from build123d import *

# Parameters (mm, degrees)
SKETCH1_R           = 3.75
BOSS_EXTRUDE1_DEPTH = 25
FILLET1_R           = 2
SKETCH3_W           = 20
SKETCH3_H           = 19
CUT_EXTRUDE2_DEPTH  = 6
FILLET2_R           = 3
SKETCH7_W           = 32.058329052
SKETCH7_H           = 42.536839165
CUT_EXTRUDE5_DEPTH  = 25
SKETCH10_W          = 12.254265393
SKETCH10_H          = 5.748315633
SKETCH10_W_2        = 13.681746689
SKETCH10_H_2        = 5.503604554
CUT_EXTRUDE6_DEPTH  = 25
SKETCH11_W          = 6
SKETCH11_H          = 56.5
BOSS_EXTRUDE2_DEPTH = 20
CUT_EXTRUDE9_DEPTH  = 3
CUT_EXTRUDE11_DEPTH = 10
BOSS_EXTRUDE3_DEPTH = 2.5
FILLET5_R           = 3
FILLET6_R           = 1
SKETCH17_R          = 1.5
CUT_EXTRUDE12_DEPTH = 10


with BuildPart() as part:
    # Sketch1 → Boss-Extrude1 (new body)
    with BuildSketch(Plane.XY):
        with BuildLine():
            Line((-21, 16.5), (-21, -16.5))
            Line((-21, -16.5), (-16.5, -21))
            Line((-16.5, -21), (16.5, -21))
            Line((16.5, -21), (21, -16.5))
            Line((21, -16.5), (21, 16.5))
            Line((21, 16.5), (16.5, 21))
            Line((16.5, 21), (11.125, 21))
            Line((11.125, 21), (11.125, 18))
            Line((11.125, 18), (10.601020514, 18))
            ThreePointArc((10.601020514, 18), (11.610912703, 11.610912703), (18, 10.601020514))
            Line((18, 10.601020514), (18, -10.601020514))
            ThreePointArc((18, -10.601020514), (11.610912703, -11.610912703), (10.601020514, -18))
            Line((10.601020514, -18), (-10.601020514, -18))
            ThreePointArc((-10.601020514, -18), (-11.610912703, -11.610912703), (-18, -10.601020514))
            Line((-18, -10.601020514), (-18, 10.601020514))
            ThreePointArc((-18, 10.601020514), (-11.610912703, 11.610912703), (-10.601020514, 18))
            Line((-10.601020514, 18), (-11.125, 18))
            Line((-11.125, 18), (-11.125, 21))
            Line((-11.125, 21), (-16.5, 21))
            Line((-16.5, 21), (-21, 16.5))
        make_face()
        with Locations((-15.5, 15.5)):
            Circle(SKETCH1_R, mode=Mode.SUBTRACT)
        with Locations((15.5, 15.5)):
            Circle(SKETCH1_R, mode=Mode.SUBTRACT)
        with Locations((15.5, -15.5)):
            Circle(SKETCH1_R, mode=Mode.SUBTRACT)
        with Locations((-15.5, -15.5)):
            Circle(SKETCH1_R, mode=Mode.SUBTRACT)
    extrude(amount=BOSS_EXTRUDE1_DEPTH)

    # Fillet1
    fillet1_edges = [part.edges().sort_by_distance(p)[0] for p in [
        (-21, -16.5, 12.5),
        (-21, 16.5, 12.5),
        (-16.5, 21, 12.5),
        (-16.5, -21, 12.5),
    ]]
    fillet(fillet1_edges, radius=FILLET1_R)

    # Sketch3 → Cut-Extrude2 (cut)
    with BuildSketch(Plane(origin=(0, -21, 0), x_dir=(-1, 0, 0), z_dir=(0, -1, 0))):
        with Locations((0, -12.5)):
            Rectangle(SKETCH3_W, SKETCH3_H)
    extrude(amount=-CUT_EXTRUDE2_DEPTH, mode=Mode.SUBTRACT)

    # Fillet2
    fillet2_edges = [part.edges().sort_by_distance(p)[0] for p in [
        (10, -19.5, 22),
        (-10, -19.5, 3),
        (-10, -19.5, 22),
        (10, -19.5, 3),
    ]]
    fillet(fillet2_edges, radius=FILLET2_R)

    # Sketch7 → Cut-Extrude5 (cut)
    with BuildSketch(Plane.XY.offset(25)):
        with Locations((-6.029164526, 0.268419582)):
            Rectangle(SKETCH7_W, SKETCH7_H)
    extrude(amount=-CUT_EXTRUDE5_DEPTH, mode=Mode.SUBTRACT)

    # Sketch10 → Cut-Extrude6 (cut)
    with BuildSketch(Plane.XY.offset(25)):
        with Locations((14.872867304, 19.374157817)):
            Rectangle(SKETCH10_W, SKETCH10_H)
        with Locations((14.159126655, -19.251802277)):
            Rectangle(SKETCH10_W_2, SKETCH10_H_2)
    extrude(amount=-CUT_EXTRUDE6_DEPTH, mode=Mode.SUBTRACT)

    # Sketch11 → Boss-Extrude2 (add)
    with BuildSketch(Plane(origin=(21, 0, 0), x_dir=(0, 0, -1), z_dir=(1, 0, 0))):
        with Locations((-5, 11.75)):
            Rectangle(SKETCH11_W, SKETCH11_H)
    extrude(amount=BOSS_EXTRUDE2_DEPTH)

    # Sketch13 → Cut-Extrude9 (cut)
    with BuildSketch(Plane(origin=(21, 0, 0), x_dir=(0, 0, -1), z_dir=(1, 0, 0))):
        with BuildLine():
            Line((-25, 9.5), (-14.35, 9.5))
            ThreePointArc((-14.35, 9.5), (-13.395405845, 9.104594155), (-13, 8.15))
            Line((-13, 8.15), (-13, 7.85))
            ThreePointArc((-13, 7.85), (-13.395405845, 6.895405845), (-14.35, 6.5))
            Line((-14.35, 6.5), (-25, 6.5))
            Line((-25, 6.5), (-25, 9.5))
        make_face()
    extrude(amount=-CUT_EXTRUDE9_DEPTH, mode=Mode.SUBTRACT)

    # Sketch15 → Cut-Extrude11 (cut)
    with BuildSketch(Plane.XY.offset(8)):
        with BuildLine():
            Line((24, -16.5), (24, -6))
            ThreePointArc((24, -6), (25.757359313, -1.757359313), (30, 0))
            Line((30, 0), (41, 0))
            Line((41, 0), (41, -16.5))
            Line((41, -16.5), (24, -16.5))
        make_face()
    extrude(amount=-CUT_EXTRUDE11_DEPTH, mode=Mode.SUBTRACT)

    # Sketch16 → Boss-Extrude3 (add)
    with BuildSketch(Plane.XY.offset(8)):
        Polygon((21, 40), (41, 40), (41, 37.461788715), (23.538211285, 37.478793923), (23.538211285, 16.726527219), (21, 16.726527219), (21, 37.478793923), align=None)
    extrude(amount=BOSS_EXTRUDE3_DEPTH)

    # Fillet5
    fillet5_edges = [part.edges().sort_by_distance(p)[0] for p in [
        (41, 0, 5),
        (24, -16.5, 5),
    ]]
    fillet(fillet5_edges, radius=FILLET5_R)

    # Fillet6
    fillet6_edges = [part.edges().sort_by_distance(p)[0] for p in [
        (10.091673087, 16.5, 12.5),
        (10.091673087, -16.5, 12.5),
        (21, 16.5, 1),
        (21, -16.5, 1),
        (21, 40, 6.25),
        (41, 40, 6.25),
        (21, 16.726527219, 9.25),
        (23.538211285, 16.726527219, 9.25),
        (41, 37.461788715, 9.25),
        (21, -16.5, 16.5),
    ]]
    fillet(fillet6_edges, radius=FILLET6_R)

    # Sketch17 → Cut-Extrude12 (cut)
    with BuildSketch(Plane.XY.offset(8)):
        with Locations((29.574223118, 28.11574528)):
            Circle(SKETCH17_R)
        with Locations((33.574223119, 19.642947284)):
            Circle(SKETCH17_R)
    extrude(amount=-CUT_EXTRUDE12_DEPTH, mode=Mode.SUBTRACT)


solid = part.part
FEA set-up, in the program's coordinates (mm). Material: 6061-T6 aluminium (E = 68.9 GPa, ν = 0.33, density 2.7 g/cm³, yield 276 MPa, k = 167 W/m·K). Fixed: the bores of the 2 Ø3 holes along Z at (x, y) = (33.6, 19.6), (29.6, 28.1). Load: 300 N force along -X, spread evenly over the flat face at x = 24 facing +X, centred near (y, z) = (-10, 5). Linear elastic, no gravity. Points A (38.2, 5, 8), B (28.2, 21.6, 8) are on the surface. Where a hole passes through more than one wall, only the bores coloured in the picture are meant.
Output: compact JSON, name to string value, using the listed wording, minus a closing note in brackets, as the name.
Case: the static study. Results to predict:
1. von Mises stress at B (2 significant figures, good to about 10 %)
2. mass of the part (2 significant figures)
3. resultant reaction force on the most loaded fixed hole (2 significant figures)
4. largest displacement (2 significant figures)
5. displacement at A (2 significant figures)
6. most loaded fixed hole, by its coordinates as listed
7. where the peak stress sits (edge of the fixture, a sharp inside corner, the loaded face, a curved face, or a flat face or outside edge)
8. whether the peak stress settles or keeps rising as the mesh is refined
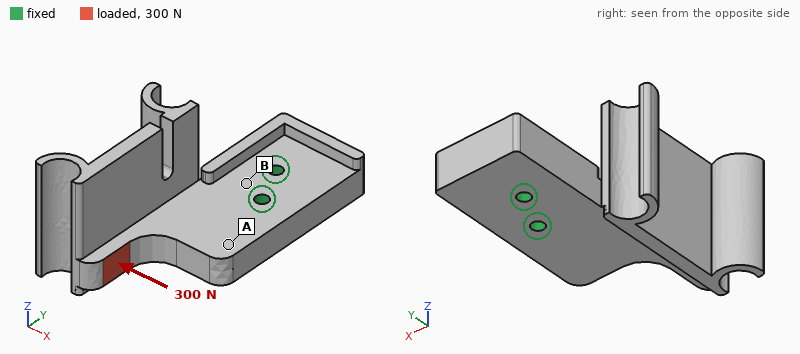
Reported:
{"von Mises stress at B": "13 MPa", "mass of the part": "23 g", "resultant reaction force on the most loaded fixed hole": "980 N", "largest displacement": "57 µm", "displacement at A": "9.9 µm", "most loaded fixed hole, by its coordinates as listed": "(33.6, 19.6)", "where the peak stress sits": "a sharp inside corner", "whether the peak stress settles or keeps rising as the mesh is refined": "keeps rising"}
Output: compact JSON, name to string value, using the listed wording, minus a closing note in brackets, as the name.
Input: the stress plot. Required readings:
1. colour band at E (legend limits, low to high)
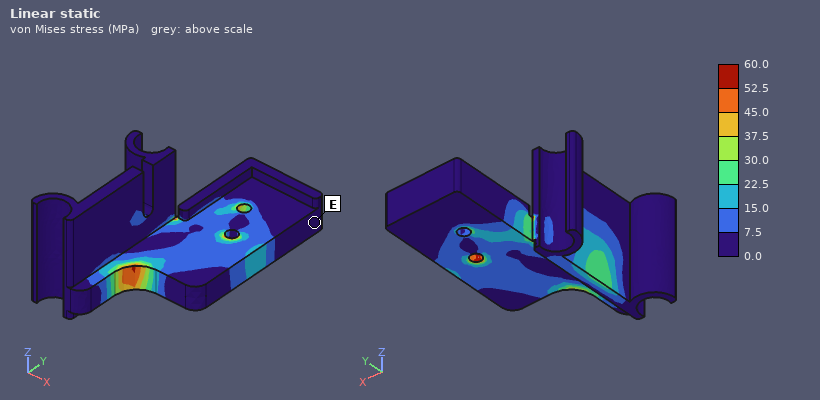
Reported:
{"colour band at E": "0.0 to 7.5 MPa"}
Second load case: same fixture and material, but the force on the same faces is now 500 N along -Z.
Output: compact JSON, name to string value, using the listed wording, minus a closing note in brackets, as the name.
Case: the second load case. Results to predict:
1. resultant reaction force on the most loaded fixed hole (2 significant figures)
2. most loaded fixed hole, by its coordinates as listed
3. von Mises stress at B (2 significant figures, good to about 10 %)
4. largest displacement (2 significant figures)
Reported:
{"resultant reaction force on the most loaded fixed hole": "970 N", "most loaded fixed hole, by its coordinates as listed": "(33.6, 19.6)", "von Mises stress at B": "63 MPa", "largest displacement": "0.32 mm"}
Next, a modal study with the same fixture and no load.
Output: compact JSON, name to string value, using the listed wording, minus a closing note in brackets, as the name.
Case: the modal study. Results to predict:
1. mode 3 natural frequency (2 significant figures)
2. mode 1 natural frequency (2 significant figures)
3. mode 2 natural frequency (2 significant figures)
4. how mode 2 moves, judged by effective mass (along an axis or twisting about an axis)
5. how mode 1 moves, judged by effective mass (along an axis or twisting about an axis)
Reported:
{"mode 3 natural frequency": "6900 Hz", "mode 1 natural frequency": "2600 Hz", "mode 2 natural frequency": "4200 Hz", "how mode 2 moves, judged by effective mass": "along X", "how mode 1 moves, judged by effective mass": "along Z"}
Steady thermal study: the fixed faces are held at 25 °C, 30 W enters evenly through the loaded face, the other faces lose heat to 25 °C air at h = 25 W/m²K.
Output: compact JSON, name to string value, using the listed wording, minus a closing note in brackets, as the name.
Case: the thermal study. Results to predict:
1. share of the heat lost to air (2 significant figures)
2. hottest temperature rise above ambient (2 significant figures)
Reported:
{"share of the heat lost to air": "11 %", "hottest temperature rise above ambient": "68 K"}
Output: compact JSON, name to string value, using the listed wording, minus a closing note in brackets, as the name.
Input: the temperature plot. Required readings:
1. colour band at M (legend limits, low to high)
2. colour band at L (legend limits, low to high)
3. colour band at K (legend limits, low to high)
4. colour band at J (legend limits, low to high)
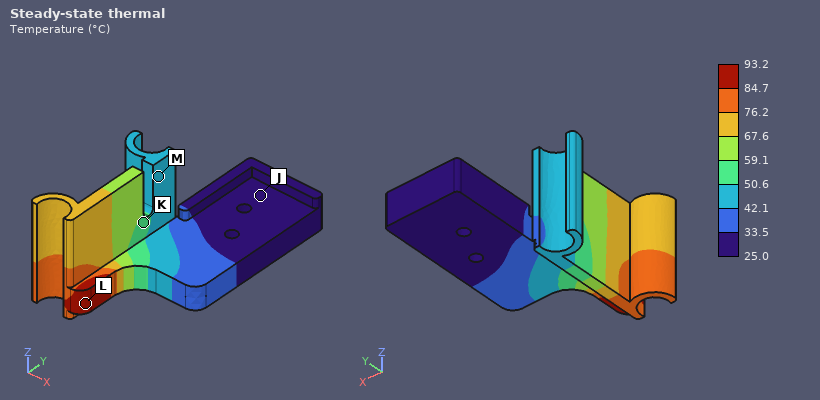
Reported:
{"colour band at M": "42.1 to 50.6 °C", "colour band at L": "84.7 to 93.2 °C", "colour band at K": "50.6 to 59.1 °C", "colour band at J": "25.0 to 33.5 °C"}
